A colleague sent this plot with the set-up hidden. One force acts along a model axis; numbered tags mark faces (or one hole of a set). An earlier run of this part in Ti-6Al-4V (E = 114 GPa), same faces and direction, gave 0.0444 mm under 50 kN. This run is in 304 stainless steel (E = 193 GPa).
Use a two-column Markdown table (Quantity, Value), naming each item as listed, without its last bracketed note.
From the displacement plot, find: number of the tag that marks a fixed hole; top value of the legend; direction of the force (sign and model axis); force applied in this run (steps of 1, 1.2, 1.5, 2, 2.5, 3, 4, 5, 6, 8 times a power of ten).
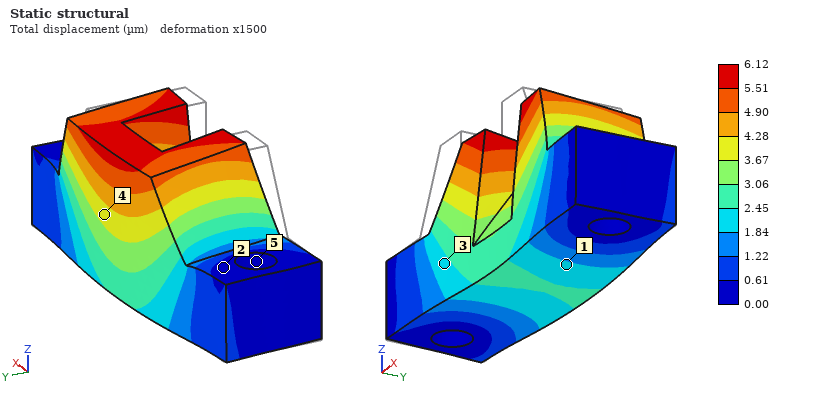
| Quantity | Value |
|---|---|
| number of the tag that marks a fixed hole | 5 |
| top value of the legend | 6.12 µm |
| direction of the force | +Y |
| force applied in this run | 12 kN |
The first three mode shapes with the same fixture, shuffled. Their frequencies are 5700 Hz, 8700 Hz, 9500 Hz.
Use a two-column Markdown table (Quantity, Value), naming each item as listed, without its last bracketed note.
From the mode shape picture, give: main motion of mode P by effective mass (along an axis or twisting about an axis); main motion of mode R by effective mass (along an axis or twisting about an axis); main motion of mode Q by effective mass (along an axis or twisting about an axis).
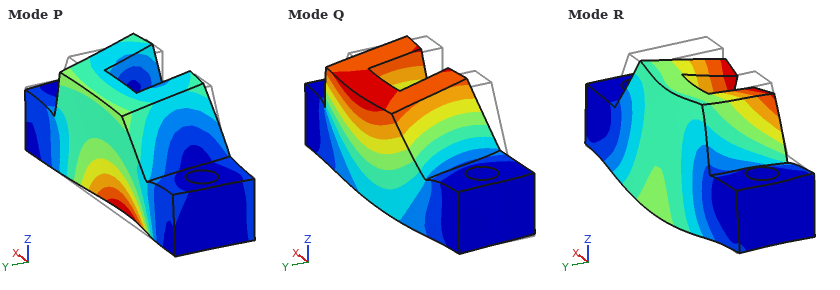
| Quantity | Value |
|---|---|
| main motion of mode P by effective mass | along Y |
| main motion of mode R by effective mass | along Z |
| main motion of mode Q by effective mass | along Y |
